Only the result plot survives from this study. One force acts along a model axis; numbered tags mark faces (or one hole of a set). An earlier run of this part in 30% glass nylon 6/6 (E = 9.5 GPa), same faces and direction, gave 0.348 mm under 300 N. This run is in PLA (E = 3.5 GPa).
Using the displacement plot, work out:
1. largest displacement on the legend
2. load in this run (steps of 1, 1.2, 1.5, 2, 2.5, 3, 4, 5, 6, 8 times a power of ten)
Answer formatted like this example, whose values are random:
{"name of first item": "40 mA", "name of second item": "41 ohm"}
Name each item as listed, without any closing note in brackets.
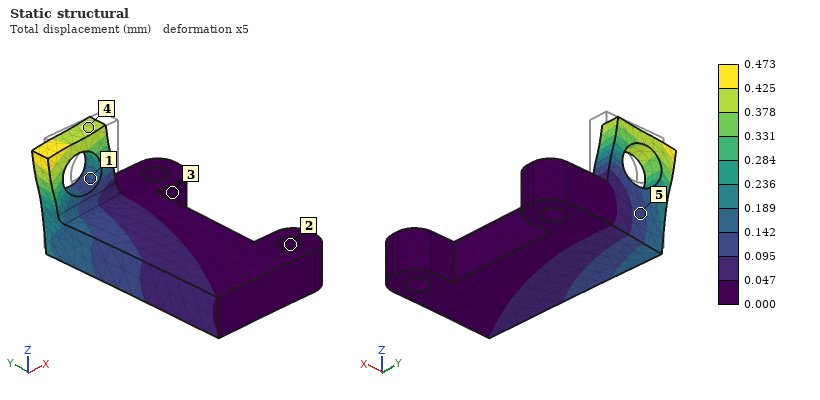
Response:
{"largest displacement on the legend": "0.473 mm", "load in this run": "150 N"}
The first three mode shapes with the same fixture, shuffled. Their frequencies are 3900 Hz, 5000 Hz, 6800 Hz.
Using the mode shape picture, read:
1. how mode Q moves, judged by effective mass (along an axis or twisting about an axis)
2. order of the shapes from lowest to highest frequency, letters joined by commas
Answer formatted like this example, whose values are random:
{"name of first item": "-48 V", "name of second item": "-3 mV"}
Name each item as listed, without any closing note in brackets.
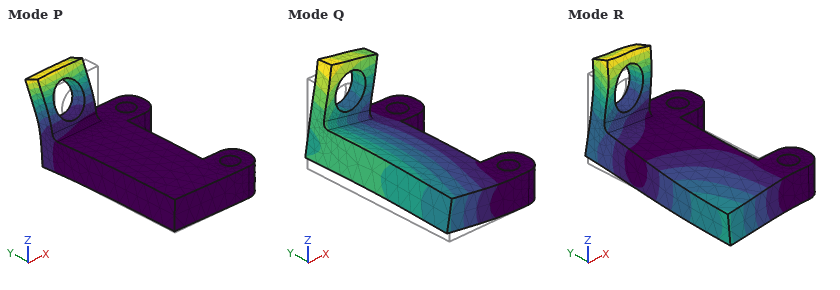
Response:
{"how mode Q moves, judged by effective mass": "along Z", "order of the shapes from lowest to highest frequency, letters joined by commas": "Q, P, R"}
